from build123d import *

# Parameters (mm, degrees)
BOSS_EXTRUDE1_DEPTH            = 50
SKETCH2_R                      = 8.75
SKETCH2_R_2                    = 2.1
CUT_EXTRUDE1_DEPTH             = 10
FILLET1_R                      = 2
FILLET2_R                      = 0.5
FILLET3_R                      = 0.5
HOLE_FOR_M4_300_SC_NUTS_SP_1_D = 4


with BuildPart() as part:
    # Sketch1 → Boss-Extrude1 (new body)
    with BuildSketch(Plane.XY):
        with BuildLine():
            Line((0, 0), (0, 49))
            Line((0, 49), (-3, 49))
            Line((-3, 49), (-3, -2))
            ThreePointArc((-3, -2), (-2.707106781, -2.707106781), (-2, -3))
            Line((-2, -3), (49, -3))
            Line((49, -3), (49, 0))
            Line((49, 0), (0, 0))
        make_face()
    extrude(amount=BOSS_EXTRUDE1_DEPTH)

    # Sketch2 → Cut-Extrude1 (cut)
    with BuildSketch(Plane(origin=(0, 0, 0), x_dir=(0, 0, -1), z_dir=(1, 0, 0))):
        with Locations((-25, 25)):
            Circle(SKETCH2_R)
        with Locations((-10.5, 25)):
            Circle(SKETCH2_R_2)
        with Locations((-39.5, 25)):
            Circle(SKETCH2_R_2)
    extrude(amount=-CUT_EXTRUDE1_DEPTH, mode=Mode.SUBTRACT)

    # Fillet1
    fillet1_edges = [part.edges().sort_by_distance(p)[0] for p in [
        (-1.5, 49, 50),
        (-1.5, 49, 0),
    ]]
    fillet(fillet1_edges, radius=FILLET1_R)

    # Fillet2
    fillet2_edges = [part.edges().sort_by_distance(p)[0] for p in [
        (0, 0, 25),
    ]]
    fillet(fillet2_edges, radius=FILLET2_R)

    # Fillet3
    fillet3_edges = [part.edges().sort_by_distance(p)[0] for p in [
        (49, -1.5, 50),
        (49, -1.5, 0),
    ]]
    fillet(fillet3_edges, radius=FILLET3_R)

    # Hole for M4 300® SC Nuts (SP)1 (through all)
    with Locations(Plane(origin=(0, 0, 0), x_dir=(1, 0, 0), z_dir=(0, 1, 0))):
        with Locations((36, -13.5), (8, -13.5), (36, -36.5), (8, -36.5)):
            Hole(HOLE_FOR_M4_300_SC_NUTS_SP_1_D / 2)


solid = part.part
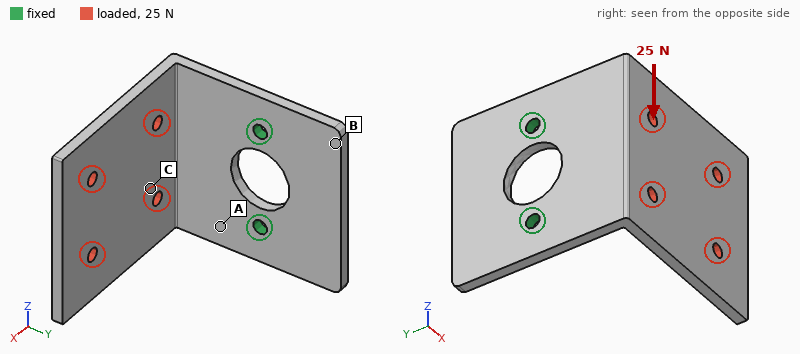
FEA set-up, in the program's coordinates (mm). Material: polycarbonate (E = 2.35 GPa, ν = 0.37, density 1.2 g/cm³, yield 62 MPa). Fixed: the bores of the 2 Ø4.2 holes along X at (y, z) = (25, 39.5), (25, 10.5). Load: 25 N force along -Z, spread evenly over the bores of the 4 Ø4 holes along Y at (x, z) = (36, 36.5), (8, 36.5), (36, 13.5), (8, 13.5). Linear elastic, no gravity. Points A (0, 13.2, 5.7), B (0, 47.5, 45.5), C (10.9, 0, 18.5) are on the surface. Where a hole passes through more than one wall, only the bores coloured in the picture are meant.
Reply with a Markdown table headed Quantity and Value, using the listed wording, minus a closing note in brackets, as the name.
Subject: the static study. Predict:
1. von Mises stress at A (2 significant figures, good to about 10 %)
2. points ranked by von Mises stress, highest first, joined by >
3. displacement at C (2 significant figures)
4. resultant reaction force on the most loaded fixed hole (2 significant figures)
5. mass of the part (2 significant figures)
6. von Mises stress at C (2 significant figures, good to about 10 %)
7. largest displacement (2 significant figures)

| Quantity | Value |
|---|---|
| von Mises stress at A | 3.3 MPa |
| points ranked by von Mises stress, highest first, joined by > | A > C > B |
| displacement at C | 0.26 mm |
| resultant reaction force on the most loaded fixed hole | 28 N |
| mass of the part | 17 g |
| von Mises stress at C | 1.3 MPa |
| largest displacement | 1.0 mm |
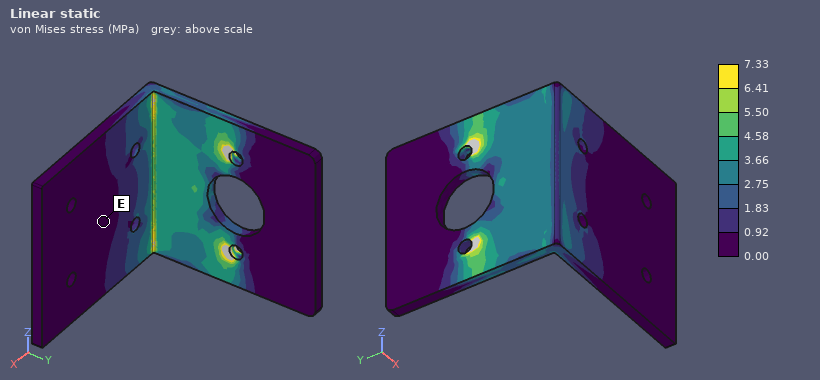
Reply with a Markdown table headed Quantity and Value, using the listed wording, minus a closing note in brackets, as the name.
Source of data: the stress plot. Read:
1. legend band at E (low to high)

| Quantity | Value |
|---|---|
| legend band at E | 0.00 to 0.92 MPa |
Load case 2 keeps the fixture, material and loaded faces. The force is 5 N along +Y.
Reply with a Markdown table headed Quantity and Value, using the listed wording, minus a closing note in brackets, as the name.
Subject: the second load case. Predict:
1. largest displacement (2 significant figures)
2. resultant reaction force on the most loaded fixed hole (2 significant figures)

| Quantity | Value |
|---|---|
| largest displacement | 0.90 mm |
| resultant reaction force on the most loaded fixed hole | 2.7 N |
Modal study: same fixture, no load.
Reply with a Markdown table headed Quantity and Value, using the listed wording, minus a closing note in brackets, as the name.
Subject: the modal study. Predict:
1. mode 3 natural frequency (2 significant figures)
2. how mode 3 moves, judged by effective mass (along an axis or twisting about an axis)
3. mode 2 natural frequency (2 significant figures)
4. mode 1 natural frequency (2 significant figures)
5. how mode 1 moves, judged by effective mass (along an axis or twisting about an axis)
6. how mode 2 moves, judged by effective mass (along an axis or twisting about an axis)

| Quantity | Value |
|---|---|
| mode 3 natural frequency | 470 Hz |
| how mode 3 moves, judged by effective mass | along X |
| mode 2 natural frequency | 290 Hz |
| mode 1 natural frequency | 140 Hz |
| how mode 1 moves, judged by effective mass | along Y |
| how mode 2 moves, judged by effective mass | along Z |
